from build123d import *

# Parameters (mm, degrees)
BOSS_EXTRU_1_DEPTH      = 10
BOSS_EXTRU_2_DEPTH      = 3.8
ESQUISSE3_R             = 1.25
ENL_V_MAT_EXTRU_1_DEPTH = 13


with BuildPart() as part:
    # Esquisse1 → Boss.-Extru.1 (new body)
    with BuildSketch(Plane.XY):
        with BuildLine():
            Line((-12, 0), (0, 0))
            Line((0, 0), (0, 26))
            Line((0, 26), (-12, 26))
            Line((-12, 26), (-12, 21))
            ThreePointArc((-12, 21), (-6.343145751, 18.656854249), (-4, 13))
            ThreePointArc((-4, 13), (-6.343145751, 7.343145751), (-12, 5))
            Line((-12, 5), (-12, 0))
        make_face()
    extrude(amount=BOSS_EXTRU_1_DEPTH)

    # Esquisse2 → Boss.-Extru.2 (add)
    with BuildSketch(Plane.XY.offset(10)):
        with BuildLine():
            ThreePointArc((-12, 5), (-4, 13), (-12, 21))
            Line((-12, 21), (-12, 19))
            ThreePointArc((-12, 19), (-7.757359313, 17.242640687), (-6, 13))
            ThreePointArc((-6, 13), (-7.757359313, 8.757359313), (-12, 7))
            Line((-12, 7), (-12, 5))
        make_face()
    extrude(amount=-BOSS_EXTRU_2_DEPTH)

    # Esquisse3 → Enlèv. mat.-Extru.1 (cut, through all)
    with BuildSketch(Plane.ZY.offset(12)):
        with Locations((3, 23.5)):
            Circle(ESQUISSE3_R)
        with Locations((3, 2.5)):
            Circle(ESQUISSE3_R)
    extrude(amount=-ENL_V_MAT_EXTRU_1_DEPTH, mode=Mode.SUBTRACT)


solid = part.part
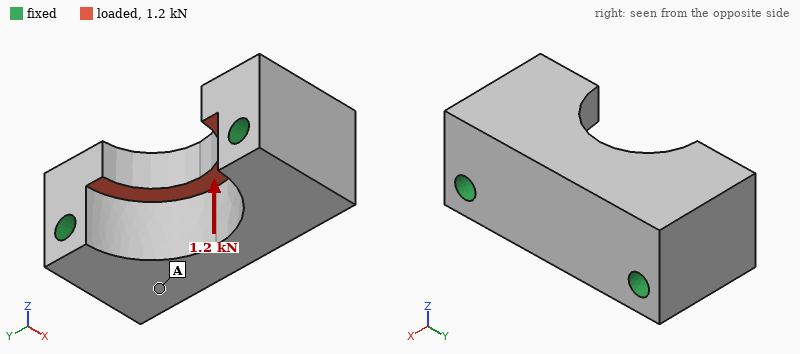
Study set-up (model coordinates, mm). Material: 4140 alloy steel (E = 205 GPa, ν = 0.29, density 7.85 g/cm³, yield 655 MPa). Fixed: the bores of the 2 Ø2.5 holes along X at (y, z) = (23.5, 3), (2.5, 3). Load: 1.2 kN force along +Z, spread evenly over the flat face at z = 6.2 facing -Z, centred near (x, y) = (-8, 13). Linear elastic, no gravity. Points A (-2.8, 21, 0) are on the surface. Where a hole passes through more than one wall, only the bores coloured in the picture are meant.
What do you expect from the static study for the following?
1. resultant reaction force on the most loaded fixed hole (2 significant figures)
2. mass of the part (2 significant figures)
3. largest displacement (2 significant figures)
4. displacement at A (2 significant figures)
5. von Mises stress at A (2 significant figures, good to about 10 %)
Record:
650 N
17 g
2.3 µm
0.40 µm
7.9 MPa
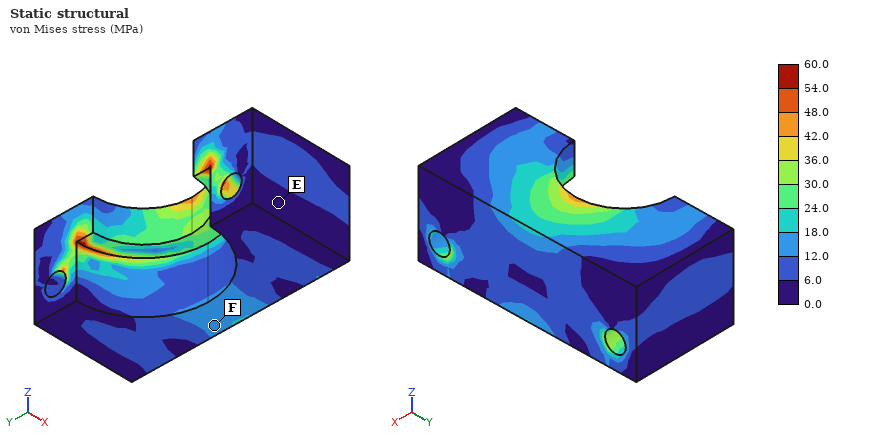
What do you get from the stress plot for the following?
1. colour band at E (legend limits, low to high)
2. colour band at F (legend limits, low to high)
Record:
0.0 to 6.0 MPa
12.0 to 18.0 MPa
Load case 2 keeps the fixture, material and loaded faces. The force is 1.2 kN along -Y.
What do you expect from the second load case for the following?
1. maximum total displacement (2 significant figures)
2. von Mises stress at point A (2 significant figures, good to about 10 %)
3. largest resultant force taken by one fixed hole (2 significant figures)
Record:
1.2 µm
4.1 MPa
620 N
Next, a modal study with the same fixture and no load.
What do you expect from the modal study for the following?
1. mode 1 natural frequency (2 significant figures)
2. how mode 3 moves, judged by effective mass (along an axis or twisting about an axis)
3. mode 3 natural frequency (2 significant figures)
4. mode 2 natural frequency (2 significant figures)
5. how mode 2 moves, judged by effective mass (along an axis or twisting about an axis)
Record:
52 kHz
along Y
72 kHz
62 kHz
along X
